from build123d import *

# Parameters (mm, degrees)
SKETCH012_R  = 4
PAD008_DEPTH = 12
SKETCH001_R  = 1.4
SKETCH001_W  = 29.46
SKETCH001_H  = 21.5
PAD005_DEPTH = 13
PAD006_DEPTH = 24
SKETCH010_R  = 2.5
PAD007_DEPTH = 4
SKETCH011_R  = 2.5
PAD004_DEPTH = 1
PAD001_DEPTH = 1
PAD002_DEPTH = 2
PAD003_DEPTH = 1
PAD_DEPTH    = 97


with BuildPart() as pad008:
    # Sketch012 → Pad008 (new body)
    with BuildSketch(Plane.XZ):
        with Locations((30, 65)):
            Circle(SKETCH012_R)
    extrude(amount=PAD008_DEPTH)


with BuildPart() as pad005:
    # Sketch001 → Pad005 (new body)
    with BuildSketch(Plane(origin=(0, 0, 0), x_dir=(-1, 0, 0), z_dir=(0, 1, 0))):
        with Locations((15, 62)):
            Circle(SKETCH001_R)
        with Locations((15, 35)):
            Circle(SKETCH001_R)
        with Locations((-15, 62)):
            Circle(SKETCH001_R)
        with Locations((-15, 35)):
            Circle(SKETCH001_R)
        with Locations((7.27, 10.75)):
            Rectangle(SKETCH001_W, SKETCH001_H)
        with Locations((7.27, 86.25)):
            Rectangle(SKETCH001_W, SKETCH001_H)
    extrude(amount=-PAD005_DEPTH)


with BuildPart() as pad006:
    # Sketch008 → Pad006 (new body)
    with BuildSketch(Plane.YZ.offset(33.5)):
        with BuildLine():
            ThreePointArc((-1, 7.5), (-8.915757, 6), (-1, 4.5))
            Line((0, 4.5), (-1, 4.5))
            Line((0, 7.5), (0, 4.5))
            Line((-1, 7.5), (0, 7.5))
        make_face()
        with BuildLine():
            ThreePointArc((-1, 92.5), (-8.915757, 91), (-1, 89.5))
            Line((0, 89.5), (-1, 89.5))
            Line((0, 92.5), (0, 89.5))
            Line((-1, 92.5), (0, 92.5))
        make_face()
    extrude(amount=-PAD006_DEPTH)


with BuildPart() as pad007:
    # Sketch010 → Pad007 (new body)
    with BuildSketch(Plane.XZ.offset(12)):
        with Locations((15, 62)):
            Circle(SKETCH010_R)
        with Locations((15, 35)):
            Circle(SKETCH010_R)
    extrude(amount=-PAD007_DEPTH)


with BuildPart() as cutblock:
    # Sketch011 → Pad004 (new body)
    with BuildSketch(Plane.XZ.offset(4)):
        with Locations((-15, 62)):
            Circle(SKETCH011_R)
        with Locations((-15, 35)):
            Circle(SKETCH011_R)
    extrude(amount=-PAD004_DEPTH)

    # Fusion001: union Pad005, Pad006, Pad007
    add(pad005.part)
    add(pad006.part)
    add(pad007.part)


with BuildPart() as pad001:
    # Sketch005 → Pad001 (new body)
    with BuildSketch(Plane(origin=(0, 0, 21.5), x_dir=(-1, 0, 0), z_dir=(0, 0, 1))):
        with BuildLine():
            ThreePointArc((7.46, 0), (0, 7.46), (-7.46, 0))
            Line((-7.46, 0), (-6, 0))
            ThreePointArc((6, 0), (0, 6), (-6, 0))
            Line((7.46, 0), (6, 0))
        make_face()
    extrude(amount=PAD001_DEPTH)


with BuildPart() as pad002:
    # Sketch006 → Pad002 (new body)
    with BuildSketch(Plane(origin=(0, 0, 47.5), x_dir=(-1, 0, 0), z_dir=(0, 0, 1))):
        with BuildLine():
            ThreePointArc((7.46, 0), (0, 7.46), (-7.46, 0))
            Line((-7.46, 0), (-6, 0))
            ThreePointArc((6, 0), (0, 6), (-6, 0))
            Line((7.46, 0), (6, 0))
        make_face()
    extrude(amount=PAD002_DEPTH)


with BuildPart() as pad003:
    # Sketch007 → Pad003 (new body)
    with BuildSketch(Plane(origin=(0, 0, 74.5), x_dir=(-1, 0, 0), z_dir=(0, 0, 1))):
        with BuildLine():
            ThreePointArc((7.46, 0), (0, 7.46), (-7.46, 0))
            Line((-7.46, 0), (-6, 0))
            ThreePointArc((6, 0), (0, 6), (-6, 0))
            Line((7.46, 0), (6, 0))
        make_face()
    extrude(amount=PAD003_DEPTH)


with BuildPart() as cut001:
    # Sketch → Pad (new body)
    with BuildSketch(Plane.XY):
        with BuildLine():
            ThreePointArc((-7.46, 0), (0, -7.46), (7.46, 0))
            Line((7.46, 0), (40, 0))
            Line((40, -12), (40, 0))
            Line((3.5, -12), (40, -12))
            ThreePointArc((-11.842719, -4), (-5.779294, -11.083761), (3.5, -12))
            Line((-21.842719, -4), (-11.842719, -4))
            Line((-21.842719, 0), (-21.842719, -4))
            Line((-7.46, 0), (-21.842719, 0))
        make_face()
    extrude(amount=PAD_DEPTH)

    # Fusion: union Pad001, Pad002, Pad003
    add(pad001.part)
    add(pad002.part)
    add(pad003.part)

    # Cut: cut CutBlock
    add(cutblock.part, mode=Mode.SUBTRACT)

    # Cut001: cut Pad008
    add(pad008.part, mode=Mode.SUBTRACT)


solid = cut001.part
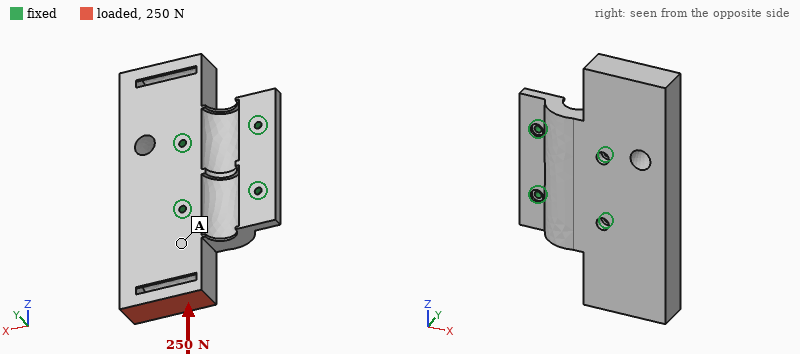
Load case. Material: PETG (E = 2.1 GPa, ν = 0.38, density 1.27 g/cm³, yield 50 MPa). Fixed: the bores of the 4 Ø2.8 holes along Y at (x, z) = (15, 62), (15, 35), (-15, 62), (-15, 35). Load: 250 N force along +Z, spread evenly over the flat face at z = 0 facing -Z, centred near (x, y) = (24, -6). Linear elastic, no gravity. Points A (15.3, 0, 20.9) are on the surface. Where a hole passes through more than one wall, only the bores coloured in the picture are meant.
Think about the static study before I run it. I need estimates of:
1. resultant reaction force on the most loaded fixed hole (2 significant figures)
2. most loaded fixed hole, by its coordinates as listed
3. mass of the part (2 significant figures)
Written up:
180 N
(15, 35)
55 g
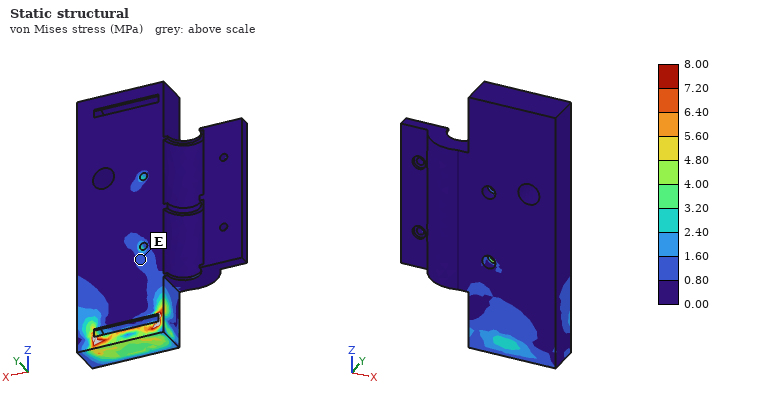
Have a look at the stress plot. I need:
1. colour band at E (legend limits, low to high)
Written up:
0.80 to 1.60 MPa
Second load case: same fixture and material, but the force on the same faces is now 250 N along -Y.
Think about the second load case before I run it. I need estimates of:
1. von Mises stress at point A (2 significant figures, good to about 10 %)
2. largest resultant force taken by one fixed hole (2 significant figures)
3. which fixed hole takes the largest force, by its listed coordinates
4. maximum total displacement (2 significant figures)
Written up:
6.7 MPa
560 N
(15, 35)
0.79 mm
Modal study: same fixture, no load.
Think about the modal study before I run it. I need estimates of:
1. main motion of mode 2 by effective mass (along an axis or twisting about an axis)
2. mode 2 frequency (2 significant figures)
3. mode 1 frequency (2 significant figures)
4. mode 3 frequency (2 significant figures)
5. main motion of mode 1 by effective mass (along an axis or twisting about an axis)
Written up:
along Y
1400 Hz
1300 Hz
2100 Hz
twisting about X
